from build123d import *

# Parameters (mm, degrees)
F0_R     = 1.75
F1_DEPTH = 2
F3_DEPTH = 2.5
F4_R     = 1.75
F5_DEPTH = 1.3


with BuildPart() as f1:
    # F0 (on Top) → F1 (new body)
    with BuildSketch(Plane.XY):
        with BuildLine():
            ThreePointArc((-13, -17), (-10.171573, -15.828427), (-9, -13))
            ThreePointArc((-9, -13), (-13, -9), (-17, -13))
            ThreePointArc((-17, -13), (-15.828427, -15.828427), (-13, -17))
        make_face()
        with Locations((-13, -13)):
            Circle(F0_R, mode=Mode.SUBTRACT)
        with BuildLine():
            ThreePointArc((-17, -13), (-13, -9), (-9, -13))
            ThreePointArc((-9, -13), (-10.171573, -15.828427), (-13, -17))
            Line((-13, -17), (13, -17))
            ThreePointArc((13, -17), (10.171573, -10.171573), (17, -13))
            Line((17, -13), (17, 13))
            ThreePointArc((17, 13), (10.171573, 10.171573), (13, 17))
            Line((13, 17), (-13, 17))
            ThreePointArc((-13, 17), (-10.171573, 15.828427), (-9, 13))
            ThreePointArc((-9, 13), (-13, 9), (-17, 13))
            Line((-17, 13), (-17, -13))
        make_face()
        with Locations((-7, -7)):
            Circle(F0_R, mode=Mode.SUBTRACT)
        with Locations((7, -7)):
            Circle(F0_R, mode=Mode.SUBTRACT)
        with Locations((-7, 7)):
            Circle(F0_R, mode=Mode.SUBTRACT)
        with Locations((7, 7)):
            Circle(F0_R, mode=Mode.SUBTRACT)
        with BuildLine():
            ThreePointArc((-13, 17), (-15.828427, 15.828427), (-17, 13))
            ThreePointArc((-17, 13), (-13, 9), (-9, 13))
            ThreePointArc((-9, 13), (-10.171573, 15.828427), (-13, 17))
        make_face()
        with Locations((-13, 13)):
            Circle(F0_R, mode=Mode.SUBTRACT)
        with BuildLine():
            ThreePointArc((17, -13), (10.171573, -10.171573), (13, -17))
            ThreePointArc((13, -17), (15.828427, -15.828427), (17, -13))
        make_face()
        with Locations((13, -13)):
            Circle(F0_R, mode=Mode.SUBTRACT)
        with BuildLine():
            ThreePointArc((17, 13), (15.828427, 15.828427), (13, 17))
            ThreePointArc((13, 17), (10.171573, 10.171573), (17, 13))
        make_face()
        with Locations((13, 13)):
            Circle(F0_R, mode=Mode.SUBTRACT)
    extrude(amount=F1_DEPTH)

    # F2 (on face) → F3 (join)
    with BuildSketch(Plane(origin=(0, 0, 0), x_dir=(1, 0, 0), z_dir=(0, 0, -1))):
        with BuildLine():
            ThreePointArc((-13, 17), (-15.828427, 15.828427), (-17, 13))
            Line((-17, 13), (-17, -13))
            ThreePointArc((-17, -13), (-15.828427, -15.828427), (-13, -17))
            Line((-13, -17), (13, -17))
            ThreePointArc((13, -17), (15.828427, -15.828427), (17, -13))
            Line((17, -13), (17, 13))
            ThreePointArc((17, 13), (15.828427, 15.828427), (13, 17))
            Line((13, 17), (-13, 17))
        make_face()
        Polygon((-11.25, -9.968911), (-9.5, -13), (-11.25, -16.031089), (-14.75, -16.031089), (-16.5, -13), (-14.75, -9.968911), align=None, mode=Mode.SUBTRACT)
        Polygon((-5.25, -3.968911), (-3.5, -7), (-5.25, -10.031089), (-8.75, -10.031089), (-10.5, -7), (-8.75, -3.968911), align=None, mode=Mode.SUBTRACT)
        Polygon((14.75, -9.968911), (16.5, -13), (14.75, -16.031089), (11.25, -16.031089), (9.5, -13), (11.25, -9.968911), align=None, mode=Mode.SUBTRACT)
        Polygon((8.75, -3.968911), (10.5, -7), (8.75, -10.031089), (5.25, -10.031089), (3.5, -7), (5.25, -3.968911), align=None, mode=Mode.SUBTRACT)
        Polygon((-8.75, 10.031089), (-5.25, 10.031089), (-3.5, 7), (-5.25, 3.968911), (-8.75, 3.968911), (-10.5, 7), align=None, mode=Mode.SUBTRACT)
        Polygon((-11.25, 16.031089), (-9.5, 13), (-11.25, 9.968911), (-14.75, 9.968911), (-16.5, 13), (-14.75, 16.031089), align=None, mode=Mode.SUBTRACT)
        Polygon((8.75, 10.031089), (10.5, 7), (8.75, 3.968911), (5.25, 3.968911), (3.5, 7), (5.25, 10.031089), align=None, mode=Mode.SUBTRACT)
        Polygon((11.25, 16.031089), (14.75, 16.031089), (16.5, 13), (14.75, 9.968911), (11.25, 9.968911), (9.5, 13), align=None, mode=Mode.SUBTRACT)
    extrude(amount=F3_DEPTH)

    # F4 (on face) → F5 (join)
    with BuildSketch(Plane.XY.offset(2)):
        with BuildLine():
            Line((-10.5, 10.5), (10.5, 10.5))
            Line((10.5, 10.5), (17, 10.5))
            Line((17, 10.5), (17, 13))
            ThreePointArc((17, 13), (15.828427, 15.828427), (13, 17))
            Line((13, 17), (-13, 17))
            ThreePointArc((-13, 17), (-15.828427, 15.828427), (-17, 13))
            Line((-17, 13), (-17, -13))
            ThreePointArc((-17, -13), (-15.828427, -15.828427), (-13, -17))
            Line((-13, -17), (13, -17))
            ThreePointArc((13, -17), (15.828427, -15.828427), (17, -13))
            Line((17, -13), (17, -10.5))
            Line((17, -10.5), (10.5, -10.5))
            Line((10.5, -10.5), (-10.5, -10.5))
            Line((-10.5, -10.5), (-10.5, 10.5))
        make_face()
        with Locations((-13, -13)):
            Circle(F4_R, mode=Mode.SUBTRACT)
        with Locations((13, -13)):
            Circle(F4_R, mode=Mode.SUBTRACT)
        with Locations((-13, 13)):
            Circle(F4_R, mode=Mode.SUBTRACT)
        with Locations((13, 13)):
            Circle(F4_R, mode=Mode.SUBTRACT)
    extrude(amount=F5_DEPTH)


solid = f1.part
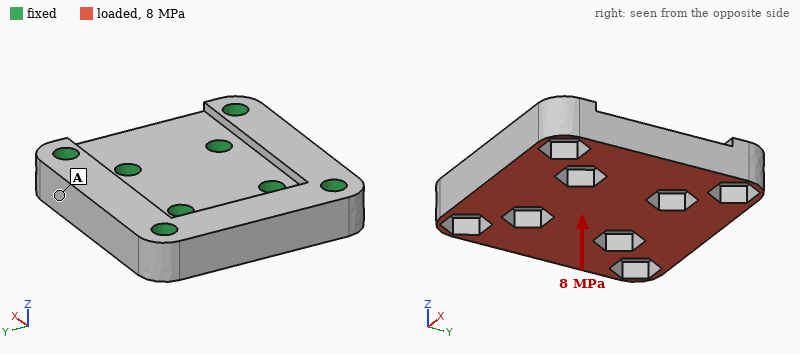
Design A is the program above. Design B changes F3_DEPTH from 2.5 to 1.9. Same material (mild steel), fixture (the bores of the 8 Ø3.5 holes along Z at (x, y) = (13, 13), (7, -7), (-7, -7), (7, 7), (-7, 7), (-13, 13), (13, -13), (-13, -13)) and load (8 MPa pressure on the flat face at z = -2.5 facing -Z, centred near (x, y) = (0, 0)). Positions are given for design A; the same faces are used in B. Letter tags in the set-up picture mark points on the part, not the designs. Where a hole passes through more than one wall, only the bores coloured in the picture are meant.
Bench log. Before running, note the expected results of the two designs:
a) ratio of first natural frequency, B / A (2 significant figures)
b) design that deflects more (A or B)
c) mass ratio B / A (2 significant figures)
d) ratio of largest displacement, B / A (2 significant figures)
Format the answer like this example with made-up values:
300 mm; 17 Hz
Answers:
0.97; B; 0.89; 1.3
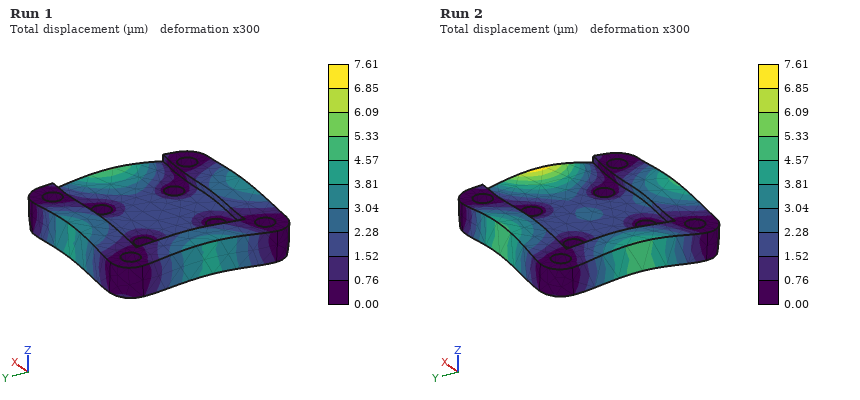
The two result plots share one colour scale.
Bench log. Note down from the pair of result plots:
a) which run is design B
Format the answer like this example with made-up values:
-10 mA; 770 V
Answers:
Run 2
